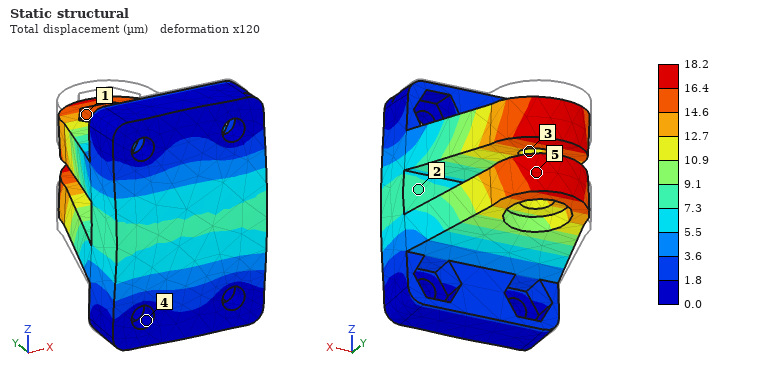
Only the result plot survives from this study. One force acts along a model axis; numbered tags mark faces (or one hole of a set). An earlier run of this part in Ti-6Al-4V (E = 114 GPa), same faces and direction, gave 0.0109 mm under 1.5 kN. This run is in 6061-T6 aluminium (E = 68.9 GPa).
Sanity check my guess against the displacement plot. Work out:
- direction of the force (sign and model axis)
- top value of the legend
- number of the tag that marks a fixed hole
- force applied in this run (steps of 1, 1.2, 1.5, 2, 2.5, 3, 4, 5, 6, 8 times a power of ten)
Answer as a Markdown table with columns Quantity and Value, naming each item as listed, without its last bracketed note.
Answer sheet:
| Quantity | Value |
|---|---|
| direction of the force | -Y |
| top value of the legend | 18.2 µm |
| number of the tag that marks a fixed hole | 4 |
| force applied in this run | 1.5 kN |
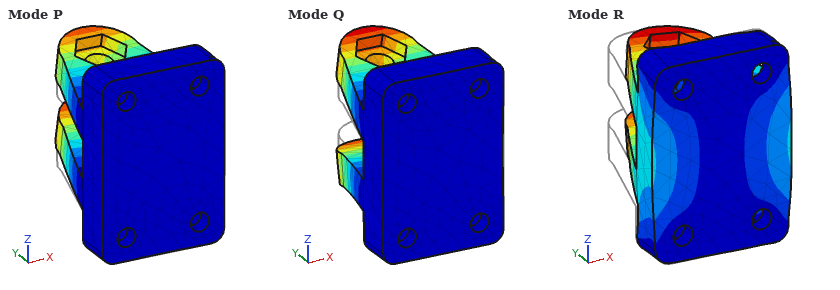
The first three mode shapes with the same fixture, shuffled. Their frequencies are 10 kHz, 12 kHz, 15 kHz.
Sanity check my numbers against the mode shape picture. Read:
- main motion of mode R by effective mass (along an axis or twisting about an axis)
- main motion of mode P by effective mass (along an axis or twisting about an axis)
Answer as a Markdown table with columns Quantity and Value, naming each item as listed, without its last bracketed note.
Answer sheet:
| Quantity | Value |
|---|---|
| main motion of mode R by effective mass | along X |
| main motion of mode P by effective mass | along Z |
